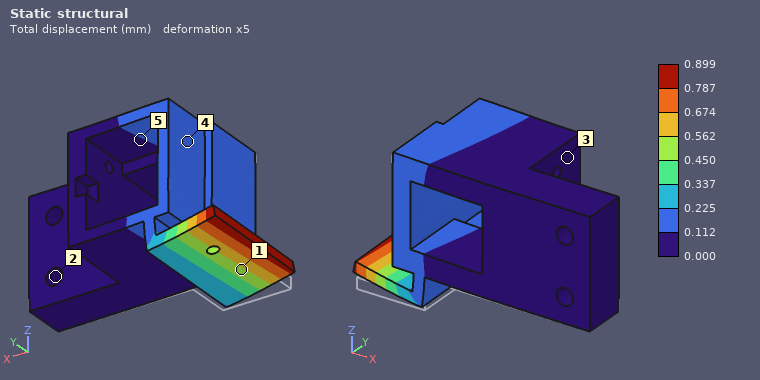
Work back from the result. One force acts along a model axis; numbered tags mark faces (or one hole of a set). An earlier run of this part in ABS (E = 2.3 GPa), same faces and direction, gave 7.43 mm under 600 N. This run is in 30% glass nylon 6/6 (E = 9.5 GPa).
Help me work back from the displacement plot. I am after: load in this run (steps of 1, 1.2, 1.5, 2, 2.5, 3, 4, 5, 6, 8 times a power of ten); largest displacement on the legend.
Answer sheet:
300 N
0.899 mm
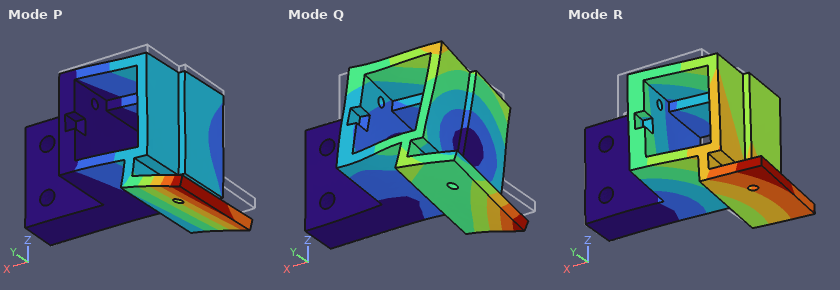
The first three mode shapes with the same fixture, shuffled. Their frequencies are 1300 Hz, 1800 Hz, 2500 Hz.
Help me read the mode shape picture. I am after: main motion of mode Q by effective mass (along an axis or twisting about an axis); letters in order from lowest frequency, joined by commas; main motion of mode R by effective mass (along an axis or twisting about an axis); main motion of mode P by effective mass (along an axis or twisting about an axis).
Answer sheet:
twisting about X
R, P, Q
along Y
along Z
